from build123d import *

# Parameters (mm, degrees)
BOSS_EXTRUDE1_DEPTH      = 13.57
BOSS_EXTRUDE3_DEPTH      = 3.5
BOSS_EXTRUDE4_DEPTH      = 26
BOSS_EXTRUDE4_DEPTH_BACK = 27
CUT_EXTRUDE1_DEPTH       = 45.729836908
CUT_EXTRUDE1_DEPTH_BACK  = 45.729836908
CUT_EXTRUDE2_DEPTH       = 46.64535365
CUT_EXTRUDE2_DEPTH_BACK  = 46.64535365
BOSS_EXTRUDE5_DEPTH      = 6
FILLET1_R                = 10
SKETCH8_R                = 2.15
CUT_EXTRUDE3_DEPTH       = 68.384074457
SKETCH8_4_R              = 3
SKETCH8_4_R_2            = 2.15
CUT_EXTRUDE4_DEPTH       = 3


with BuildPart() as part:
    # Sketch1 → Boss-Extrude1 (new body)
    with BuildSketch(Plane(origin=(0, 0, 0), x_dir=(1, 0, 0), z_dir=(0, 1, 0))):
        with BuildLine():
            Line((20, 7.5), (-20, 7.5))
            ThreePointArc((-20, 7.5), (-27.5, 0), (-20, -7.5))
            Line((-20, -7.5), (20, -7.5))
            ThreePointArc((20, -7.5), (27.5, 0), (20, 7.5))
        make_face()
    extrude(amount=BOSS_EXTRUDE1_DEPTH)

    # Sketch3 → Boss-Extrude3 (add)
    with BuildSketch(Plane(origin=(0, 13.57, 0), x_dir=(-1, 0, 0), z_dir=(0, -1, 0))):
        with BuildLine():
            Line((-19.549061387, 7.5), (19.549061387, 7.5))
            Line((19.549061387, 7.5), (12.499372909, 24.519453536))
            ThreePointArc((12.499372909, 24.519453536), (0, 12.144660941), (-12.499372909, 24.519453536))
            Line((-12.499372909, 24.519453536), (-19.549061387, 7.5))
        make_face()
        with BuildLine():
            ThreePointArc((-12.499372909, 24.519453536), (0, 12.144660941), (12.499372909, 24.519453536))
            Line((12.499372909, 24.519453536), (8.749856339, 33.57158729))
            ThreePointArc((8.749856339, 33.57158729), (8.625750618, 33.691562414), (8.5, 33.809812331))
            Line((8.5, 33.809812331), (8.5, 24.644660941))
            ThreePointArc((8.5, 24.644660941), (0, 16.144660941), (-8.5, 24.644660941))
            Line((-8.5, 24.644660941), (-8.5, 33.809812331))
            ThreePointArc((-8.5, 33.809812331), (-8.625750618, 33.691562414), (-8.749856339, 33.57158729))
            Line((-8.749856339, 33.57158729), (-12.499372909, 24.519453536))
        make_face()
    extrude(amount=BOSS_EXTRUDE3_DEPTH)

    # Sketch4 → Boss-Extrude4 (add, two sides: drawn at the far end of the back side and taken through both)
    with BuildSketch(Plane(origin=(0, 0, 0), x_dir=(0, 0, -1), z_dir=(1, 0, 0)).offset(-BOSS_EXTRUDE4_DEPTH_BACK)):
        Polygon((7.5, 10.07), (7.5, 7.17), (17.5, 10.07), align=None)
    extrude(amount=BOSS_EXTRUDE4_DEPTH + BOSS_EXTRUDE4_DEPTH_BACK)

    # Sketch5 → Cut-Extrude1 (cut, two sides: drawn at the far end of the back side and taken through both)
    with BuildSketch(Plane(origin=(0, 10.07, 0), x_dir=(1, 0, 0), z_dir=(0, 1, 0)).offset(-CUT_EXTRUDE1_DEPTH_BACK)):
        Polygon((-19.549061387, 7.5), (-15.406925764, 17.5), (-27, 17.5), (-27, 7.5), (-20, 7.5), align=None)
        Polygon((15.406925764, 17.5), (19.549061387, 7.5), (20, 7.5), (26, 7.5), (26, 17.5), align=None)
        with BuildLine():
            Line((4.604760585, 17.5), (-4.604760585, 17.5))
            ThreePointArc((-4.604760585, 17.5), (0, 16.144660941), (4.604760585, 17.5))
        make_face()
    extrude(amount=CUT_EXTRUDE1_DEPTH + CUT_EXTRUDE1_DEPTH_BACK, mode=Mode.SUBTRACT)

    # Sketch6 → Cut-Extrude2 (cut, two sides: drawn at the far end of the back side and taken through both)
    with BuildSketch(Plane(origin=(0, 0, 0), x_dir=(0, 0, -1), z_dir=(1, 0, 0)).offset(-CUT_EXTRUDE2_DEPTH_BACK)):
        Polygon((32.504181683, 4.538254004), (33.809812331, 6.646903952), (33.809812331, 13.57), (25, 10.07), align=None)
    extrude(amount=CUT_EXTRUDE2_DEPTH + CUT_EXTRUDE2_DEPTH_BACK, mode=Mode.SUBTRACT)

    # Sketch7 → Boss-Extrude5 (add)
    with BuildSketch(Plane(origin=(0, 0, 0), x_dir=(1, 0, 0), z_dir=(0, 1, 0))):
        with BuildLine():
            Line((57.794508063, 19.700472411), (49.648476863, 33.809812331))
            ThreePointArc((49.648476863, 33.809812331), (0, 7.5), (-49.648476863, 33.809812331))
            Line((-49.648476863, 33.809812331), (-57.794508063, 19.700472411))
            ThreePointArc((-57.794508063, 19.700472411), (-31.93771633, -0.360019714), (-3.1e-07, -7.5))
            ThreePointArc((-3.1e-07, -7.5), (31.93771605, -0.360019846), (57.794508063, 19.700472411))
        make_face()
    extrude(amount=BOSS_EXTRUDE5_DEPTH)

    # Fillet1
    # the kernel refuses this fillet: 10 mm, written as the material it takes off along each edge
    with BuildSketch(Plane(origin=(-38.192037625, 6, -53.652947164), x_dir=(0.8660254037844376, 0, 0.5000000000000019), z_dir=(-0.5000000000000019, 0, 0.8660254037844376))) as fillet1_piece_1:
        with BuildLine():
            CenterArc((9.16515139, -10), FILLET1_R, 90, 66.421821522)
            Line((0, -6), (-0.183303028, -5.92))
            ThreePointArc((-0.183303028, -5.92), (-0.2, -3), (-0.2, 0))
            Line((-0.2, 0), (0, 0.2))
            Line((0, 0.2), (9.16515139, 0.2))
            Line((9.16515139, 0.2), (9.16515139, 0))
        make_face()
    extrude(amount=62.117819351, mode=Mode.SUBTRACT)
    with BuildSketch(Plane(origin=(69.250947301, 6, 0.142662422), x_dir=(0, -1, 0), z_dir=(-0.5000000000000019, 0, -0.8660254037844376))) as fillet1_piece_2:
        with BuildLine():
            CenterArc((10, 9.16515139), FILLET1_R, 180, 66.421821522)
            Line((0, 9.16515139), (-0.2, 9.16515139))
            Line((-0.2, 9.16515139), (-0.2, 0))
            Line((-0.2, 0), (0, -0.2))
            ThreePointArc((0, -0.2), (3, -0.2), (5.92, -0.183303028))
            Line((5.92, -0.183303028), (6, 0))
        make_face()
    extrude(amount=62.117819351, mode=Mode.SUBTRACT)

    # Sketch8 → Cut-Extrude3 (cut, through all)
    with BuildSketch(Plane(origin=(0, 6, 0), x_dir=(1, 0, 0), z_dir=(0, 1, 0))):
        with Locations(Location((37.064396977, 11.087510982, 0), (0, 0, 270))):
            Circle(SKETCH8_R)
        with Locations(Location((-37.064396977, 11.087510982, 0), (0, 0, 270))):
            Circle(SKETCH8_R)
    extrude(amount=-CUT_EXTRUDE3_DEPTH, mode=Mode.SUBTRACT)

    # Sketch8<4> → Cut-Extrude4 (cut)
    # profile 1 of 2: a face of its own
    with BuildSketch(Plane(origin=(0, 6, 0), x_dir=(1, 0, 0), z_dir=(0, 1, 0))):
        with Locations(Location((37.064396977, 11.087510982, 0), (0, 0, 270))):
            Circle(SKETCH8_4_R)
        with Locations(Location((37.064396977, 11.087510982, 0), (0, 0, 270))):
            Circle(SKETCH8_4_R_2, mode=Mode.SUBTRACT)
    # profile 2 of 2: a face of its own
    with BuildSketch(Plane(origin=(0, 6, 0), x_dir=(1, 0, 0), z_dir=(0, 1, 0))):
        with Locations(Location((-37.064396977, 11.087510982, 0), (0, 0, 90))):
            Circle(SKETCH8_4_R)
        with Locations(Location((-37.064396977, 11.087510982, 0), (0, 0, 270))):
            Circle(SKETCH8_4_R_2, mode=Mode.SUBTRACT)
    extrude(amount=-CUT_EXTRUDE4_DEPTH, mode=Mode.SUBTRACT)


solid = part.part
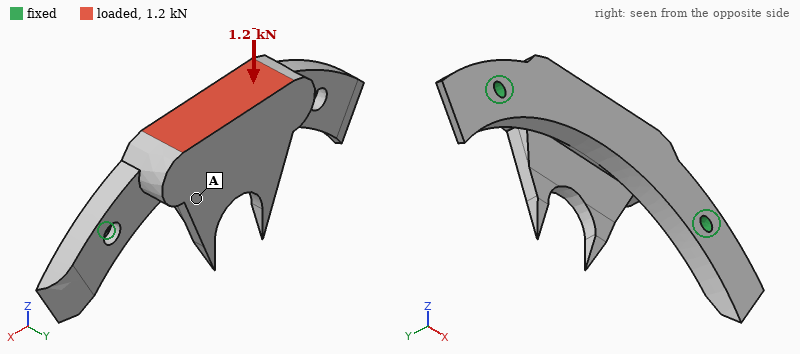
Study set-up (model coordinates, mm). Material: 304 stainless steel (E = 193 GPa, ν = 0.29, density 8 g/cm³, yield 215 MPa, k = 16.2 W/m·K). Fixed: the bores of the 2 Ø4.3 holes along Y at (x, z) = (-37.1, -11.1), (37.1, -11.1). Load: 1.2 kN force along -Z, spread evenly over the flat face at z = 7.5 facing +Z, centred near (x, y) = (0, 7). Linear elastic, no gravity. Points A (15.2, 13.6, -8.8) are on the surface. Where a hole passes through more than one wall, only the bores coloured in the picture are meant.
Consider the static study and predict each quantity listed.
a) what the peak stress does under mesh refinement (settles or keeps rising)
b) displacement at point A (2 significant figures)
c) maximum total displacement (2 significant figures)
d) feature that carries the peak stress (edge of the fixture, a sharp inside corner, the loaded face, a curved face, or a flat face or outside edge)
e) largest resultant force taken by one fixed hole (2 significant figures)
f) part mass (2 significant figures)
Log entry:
keeps rising
14 µm
26 µm
edge of the fixture
840 N
150 g
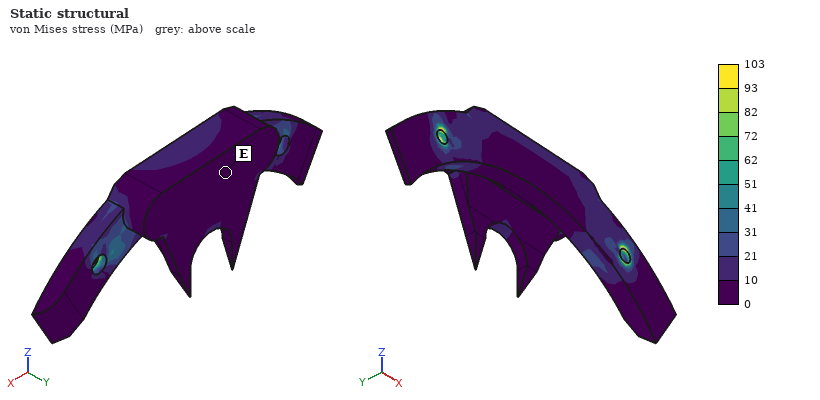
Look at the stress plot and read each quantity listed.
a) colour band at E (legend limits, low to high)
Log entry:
0 to 10 MPa
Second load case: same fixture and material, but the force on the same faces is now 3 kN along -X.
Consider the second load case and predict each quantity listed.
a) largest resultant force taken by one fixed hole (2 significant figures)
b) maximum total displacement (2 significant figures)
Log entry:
1.7 kN
3.8 µm
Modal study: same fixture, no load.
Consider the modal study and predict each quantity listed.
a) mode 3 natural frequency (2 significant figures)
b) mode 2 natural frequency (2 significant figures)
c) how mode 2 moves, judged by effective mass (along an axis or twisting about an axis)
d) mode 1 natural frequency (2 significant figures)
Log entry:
7800 Hz
5900 Hz
along Y
3000 Hz
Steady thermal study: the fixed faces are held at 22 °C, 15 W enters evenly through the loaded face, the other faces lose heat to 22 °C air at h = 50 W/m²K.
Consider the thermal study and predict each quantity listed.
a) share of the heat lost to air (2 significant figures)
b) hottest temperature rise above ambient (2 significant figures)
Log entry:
64 %
65 K
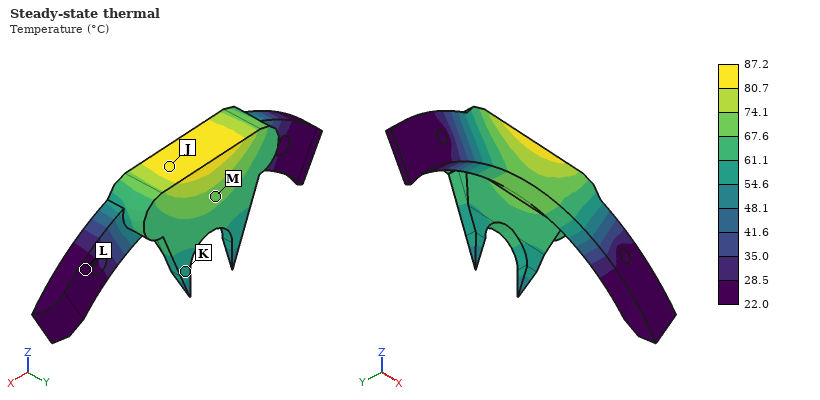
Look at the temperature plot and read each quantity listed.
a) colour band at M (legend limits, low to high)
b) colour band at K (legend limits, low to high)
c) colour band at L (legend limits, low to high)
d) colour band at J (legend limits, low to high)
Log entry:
67.6 to 74.1 °C
54.6 to 61.1 °C
22.0 to 28.5 °C
80.7 to 87.2 °C
